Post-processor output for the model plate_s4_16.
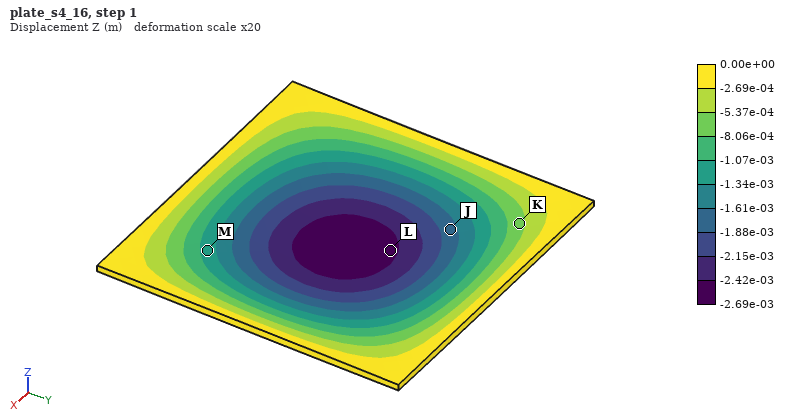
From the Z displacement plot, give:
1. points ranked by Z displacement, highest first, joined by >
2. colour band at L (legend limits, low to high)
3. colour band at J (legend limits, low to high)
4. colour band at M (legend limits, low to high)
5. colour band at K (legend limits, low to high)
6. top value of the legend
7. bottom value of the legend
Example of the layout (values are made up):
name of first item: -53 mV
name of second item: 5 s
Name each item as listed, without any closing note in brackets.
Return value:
points ranked by Z displacement, highest first, joined by >: K > M > J > L
colour band at L: -2.69e-03 to -2.42e-03 m
colour band at J: -1.88e-03 to -1.61e-03 m
colour band at M: -1.34e-03 to -1.07e-03 m
colour band at K: -8.06e-04 to -5.37e-04 m
top value of the legend: 0.00e+00 m
bottom value of the legend: -2.69e-03 m
